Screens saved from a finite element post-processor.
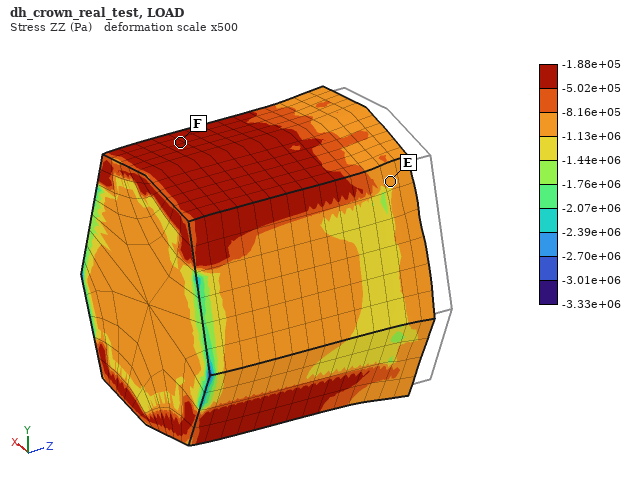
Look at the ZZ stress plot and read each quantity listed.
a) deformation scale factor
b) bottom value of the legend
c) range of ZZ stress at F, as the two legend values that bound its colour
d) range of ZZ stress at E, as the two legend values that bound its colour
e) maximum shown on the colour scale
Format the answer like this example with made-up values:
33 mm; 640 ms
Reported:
500; -3.33e+06 Pa; -5.02e+05 to -1.88e+05 Pa; -1.13e+06 to -8.16e+05 Pa; -1.88e+05 Pa
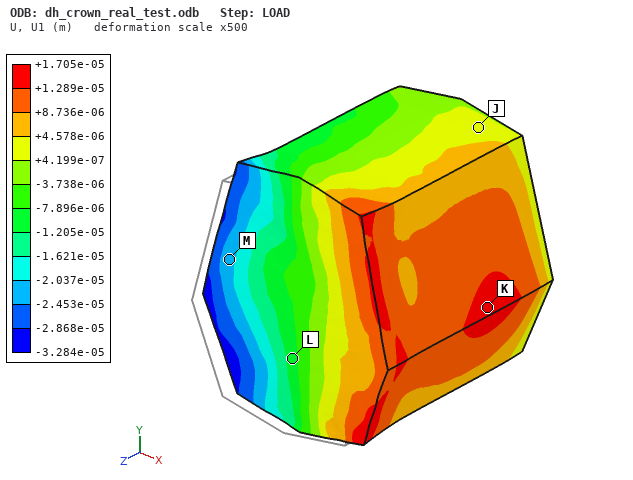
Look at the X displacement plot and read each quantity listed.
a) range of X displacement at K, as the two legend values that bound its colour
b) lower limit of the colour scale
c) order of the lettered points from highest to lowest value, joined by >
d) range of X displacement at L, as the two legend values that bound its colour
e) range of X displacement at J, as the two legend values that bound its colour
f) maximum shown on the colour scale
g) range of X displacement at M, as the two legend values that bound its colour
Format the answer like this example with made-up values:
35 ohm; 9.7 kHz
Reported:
+1.289e-05 to +1.705e-05 m; -3.284e-05 m; K > J > L > M; -1.205e-05 to -7.896e-06 m; +4.199e-07 to +4.578e-06 m; +1.705e-05 m; -2.453e-05 to -2.037e-05 m
